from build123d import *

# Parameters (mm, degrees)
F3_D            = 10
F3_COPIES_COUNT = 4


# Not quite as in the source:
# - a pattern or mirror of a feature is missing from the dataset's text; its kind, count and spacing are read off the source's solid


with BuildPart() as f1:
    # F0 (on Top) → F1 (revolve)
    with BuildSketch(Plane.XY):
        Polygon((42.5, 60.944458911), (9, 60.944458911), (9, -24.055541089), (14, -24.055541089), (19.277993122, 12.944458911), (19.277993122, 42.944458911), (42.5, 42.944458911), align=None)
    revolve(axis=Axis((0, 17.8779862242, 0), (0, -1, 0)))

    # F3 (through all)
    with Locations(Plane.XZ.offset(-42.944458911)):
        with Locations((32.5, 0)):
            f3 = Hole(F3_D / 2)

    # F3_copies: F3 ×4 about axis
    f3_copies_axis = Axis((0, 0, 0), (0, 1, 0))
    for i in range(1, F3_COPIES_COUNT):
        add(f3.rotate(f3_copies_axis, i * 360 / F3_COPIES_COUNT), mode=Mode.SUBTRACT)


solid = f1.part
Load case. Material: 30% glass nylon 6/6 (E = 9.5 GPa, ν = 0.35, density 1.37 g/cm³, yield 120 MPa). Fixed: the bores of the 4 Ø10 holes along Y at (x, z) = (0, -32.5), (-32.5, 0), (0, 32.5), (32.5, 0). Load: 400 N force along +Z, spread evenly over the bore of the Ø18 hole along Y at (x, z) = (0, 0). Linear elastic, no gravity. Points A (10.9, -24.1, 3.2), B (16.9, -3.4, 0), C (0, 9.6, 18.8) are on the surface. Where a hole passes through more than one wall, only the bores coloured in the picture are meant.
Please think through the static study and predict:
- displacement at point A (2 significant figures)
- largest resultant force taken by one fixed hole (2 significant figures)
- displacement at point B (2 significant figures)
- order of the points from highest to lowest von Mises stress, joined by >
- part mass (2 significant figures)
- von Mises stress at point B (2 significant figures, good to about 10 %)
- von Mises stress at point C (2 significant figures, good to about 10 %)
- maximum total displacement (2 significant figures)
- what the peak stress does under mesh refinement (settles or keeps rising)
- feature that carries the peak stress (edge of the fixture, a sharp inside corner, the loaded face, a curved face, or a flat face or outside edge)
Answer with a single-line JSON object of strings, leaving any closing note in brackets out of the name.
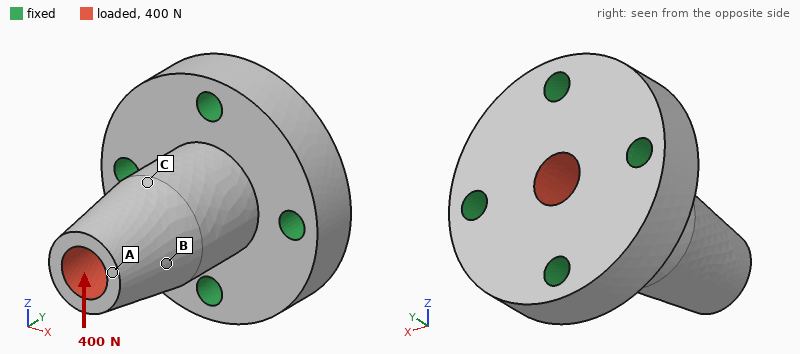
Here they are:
{"displacement at point A": "28 µm", "largest resultant force taken by one fixed hole": "260 N", "displacement at point B": "19 µm", "order of the points from highest to lowest von Mises stress, joined by >": "C > B > A", "part mass": "190 g", "von Mises stress at point B": "0.39 MPa", "von Mises stress at point C": "0.55 MPa", "maximum total displacement": "29 µm", "what the peak stress does under mesh refinement": "keeps rising", "feature that carries the peak stress": "edge of the fixture"}
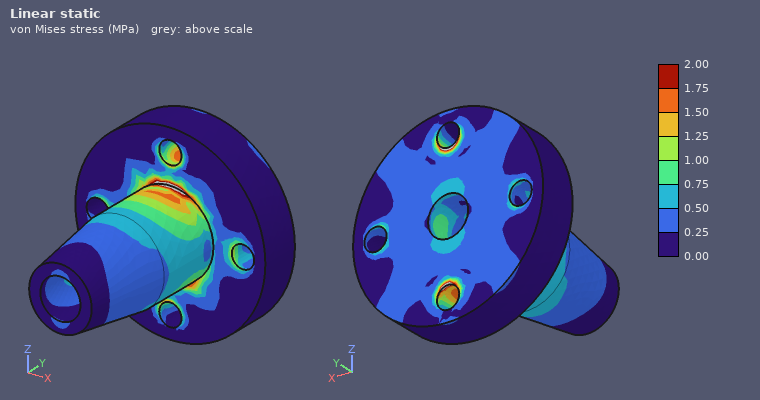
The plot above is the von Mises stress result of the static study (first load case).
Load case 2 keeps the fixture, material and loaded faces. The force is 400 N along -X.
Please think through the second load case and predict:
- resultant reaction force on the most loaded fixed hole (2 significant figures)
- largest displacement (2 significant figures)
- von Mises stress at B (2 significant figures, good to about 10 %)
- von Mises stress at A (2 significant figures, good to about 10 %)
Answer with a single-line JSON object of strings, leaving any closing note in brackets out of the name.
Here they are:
{"resultant reaction force on the most loaded fixed hole": "260 N", "largest displacement": "29 µm", "von Mises stress at B": "0.34 MPa", "von Mises stress at A": "0.24 MPa"}
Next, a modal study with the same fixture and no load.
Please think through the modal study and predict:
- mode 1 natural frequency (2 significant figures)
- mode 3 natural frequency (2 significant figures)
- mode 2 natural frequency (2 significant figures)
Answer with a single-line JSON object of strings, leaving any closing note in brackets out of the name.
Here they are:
{"mode 1 natural frequency": "2800 Hz", "mode 3 natural frequency": "6900 Hz", "mode 2 natural frequency": "2800 Hz"}
